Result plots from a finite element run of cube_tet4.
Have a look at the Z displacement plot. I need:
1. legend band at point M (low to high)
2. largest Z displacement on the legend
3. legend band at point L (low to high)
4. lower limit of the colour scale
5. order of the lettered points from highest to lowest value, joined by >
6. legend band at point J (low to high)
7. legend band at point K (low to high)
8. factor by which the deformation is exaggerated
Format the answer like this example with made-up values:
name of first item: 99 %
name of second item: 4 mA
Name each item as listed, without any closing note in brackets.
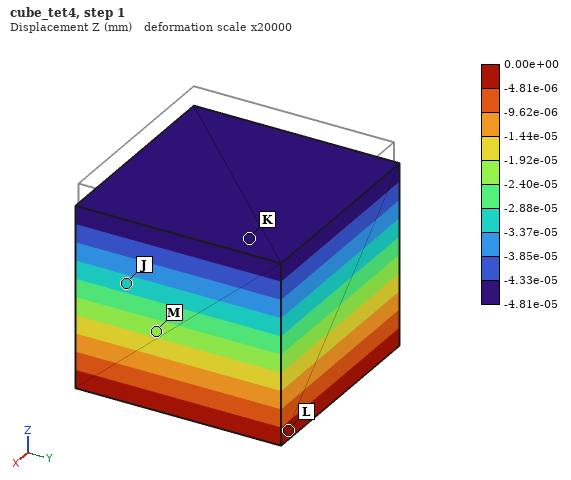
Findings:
legend band at point M: -2.40e-05 to -1.92e-05 mm
largest Z displacement on the legend: 0.00e+00 mm
legend band at point L: -4.81e-06 to 0.00e+00 mm
lower limit of the colour scale: -4.81e-05 mm
order of the lettered points from highest to lowest value, joined by >: L > M > J > K
legend band at point J: -3.37e-05 to -2.88e-05 mm
legend band at point K: -4.81e-05 to -4.33e-05 mm
factor by which the deformation is exaggerated: 20000
